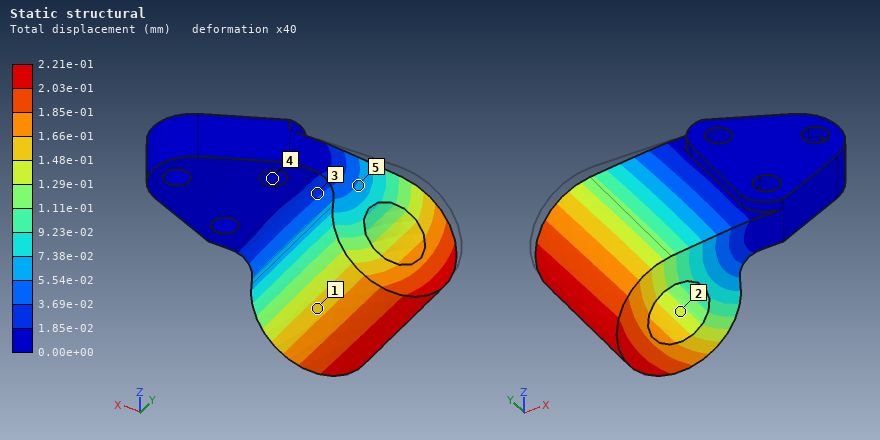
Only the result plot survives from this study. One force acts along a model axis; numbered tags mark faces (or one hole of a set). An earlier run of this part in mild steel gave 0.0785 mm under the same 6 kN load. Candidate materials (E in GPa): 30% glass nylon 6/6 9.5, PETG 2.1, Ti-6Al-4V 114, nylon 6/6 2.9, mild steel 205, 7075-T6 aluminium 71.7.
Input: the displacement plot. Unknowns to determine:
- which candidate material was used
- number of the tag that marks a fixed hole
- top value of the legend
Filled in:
7075-T6 aluminium
4
2.21e-01 mm
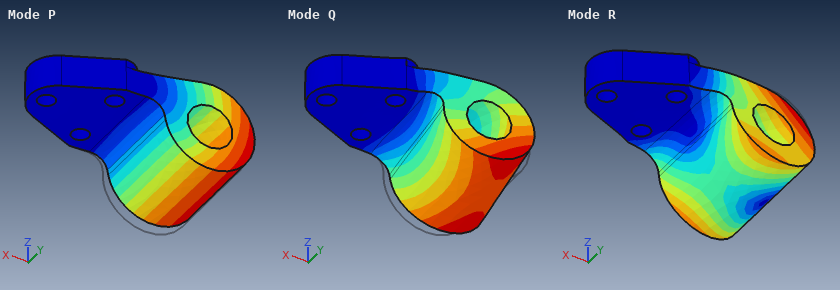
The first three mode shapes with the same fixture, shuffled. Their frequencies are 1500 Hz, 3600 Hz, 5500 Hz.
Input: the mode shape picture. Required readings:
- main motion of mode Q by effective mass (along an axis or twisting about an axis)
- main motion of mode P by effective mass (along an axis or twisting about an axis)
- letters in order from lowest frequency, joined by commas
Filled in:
along Y
along Z
P, Q, R
